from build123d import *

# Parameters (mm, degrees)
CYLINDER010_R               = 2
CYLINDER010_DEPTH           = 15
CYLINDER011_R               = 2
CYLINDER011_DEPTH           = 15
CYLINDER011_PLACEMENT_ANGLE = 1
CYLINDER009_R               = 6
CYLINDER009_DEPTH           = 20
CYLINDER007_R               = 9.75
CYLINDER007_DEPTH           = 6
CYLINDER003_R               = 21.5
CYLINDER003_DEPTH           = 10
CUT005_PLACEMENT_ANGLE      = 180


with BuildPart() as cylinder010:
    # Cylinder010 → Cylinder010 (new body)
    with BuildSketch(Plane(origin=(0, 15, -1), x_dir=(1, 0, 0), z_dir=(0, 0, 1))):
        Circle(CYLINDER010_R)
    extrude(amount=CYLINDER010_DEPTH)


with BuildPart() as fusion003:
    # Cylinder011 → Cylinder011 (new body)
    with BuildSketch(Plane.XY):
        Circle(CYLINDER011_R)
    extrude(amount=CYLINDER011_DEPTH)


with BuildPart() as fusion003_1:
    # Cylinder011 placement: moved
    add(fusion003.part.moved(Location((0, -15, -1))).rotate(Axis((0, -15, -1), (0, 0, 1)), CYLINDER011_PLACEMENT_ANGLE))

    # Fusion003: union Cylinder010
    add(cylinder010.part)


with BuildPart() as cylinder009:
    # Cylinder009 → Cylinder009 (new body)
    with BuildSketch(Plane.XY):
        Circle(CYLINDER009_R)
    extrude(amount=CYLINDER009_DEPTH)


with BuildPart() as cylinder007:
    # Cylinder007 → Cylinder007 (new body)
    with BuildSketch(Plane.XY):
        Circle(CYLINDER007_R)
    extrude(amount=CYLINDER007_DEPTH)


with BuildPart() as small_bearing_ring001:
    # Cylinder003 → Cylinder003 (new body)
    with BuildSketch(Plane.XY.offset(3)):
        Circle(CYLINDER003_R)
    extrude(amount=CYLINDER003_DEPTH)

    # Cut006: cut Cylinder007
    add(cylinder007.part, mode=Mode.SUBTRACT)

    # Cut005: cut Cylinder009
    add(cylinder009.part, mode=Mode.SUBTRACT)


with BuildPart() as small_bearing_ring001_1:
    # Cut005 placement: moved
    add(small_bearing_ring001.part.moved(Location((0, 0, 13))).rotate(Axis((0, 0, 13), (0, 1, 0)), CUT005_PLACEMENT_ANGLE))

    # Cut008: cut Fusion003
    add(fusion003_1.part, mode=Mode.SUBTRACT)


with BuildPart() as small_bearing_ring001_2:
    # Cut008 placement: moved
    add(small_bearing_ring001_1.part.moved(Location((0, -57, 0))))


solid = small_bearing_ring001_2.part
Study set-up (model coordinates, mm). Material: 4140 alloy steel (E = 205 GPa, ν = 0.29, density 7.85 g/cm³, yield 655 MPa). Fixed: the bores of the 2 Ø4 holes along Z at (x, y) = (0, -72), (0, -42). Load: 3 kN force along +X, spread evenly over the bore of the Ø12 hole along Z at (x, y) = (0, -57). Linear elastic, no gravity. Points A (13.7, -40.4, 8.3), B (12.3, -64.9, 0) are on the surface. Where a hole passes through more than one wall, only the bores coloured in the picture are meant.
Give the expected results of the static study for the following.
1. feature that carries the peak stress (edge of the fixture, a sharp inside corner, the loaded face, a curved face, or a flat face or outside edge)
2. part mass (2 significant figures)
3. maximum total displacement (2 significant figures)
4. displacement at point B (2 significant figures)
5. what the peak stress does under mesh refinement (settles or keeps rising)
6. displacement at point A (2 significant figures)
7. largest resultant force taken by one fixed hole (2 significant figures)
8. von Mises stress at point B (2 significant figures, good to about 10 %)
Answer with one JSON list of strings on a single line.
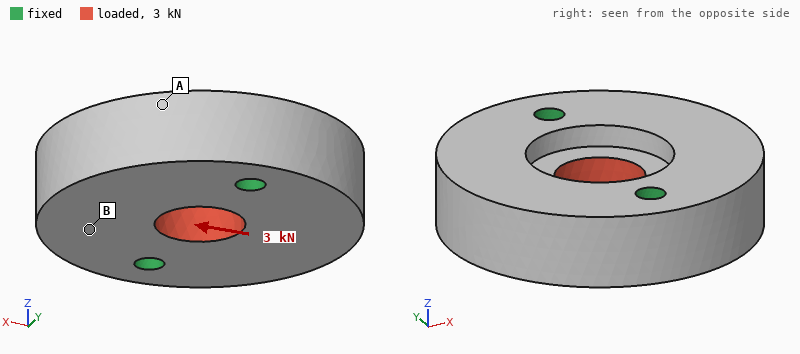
["edge of the fixture", "99 g", "1.4 µm", "1.0 µm", "keeps rising", "0.50 µm", "1.5 kN", "7.6 MPa"]
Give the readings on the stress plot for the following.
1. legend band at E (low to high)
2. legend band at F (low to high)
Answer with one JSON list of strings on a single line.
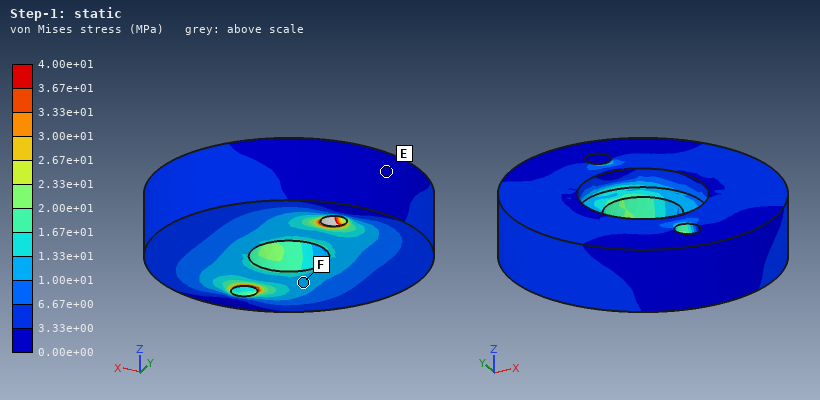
["0.00e+00 to 3.33e+00 MPa", "1.00e+01 to 1.33e+01 MPa"]
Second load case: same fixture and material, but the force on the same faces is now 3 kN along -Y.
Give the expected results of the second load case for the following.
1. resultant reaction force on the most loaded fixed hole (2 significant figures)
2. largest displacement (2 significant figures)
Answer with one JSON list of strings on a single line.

["1.5 kN", "0.97 µm"]
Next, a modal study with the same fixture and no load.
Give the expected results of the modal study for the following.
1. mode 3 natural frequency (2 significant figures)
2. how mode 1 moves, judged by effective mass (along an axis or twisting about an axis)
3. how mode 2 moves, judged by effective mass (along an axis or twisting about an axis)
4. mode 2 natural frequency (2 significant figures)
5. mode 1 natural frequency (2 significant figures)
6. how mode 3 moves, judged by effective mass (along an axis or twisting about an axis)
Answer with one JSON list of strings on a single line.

["30 kHz", "twisting about Y", "along Z", "16 kHz", "14 kHz", "twisting about Z"]
